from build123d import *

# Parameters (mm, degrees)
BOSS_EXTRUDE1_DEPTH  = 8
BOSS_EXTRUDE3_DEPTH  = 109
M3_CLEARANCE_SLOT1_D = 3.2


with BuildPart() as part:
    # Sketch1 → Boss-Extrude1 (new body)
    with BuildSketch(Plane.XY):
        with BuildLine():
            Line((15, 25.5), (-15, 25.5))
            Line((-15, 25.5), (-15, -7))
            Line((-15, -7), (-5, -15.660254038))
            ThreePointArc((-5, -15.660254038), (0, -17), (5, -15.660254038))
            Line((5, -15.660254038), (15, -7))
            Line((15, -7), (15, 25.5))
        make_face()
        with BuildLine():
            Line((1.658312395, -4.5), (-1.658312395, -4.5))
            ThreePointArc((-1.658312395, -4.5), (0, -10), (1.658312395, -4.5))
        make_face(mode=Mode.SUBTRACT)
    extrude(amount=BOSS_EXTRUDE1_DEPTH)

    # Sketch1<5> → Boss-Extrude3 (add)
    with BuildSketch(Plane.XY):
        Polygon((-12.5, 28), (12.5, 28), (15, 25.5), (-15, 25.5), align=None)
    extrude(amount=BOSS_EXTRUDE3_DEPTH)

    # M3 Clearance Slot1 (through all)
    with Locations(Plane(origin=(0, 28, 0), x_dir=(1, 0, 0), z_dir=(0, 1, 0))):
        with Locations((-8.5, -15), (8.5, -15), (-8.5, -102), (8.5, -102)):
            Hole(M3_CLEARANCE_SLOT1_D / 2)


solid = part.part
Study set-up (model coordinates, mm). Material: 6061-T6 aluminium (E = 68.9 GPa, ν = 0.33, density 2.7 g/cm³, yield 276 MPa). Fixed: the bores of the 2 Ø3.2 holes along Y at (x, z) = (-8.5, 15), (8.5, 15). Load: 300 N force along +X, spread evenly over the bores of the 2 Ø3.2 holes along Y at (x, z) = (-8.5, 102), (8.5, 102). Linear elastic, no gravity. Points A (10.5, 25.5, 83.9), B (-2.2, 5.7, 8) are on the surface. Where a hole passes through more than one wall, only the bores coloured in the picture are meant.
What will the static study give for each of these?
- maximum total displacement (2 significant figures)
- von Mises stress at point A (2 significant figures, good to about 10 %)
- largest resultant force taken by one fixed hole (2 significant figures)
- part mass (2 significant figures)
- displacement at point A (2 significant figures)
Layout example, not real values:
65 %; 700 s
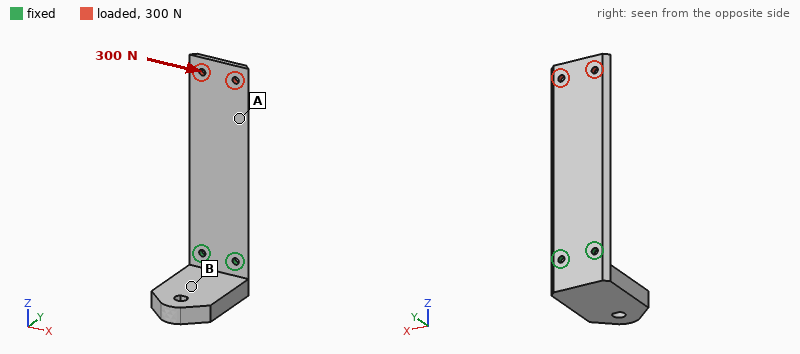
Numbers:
0.28 mm; 14 MPa; 1.4 kN; 44 g; 0.18 mm
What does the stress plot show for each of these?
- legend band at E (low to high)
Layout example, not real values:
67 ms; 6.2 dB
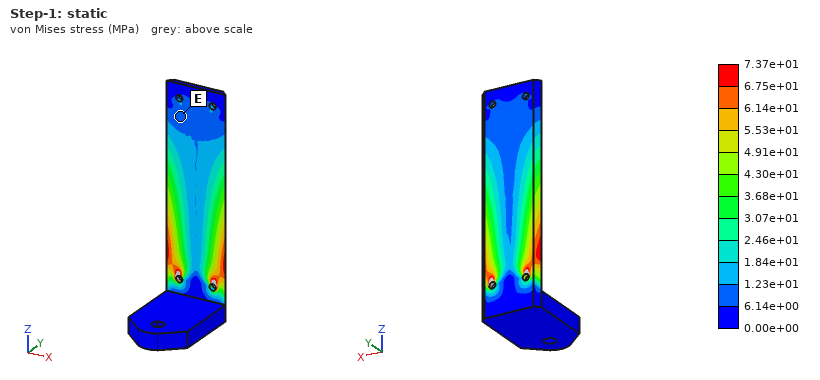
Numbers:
6.14e+00 to 1.23e+01 MPa
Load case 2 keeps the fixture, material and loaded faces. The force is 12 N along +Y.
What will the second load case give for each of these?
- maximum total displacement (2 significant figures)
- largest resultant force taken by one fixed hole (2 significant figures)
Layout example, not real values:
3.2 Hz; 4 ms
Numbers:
1.2 mm; 8.4 N
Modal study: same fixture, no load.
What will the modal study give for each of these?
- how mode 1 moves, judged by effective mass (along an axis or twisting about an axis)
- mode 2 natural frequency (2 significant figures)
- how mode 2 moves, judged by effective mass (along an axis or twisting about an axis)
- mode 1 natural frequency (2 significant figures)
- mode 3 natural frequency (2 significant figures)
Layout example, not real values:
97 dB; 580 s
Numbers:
along Y; 750 Hz; along Z; 240 Hz; 1500 Hz
